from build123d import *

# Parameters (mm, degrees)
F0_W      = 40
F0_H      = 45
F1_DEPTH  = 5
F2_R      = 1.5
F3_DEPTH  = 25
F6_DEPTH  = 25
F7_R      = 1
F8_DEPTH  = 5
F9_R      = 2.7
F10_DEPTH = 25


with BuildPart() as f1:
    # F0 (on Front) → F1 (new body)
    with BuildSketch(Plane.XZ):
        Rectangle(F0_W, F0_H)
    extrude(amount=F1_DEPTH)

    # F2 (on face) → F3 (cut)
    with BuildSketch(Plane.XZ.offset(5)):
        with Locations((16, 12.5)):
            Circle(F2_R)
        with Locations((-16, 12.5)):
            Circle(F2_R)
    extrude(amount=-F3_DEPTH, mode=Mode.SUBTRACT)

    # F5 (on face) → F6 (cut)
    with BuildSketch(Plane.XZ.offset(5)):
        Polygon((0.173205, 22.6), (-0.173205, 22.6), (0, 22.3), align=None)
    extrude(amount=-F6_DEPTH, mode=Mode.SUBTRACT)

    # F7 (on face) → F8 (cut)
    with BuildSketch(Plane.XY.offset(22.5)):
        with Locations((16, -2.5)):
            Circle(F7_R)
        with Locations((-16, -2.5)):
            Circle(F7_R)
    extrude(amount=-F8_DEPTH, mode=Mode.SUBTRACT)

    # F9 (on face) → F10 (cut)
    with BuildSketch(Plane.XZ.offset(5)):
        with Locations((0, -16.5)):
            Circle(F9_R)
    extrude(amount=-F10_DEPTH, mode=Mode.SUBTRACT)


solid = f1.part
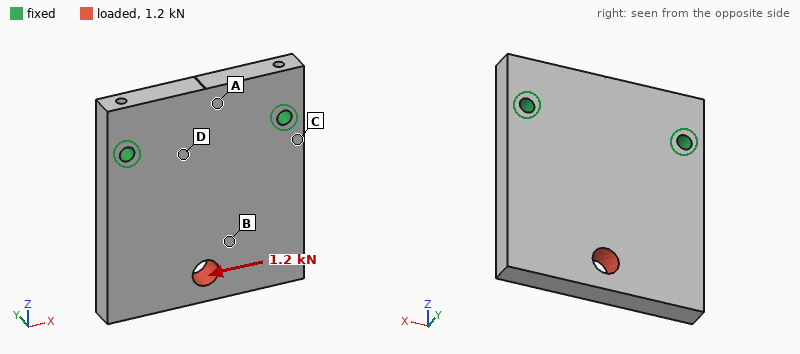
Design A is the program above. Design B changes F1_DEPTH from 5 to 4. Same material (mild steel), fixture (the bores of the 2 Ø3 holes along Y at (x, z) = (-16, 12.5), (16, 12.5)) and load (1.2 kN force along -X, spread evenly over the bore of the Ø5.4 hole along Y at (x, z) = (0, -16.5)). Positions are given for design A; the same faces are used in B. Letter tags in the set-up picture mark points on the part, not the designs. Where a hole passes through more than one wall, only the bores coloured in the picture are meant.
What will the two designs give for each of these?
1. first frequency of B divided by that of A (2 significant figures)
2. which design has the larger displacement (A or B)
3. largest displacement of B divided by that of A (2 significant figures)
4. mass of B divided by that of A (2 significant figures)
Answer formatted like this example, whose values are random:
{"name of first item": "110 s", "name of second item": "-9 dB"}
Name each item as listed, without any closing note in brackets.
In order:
{"first frequency of B divided by that of A": "0.82", "which design has the larger displacement": "B", "largest displacement of B divided by that of A": "1.3", "mass of B divided by that of A": "0.80"}
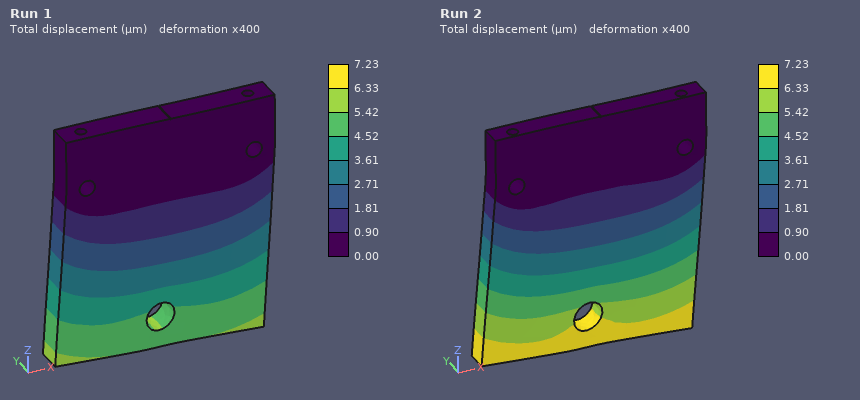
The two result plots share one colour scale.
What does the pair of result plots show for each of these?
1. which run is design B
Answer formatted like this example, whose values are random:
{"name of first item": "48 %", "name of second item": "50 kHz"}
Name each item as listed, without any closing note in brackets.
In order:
{"which run is design B": "Run 2"}
